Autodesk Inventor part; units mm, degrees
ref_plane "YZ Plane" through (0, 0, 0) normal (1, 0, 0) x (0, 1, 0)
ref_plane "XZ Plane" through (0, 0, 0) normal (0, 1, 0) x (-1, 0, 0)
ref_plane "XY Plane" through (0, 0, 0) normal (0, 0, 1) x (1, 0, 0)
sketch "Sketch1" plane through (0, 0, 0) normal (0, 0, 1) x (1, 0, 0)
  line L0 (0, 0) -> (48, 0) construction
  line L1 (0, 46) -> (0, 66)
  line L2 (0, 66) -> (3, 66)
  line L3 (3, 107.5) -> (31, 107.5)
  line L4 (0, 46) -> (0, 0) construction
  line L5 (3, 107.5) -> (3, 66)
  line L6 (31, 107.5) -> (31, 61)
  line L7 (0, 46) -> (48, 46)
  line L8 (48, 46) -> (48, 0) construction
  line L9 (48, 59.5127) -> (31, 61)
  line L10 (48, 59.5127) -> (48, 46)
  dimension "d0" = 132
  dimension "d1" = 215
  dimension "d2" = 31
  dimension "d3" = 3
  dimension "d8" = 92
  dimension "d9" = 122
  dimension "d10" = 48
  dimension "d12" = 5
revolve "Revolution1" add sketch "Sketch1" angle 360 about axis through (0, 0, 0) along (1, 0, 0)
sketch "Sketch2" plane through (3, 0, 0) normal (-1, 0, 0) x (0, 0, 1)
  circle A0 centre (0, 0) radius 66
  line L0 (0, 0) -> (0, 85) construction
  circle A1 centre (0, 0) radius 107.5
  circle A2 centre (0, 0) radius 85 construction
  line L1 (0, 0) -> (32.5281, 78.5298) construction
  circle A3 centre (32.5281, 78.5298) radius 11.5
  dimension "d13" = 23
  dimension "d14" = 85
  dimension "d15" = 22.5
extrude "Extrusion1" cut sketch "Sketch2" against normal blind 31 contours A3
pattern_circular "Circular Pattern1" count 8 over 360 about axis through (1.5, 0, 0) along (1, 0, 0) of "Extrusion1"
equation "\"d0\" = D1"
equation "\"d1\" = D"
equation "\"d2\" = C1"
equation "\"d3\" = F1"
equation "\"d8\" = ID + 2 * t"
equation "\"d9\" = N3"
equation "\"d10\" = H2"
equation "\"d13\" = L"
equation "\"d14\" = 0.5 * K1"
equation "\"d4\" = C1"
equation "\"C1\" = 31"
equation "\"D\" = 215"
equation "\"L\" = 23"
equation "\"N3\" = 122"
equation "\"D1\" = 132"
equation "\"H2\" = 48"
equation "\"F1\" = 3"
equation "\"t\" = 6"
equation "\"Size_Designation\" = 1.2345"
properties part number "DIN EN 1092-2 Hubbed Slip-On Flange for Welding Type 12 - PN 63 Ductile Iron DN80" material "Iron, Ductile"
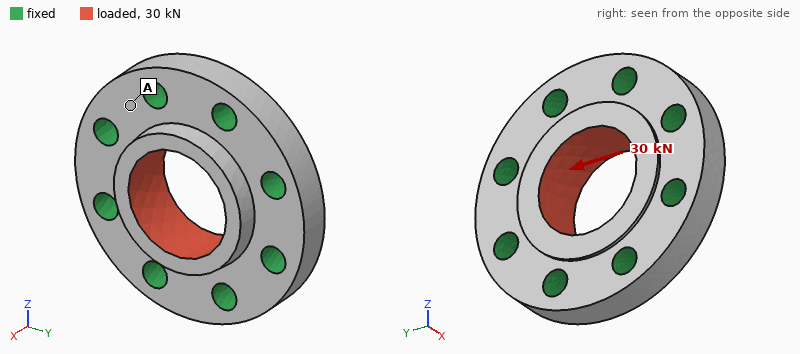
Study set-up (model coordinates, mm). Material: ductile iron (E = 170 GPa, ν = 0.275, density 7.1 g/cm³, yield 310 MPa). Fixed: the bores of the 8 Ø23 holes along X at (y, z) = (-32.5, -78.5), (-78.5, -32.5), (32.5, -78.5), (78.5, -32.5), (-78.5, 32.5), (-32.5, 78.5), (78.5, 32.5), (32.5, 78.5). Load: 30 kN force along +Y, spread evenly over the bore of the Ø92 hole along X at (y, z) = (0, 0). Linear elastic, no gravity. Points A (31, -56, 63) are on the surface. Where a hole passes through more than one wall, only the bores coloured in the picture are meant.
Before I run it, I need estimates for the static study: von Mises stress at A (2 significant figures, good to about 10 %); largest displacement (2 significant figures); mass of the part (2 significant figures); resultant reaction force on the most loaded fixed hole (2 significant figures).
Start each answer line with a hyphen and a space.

- 1.1 MPa
- 2.6 µm
- 6.0 kg
- 5.1 kN
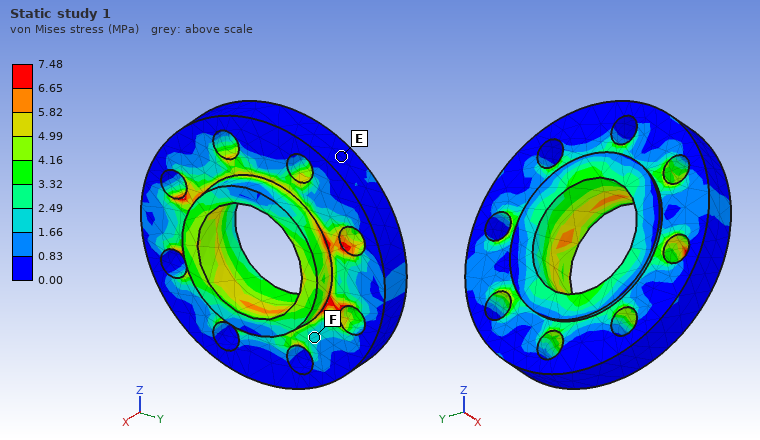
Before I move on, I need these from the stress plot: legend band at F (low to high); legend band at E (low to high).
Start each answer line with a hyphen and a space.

- 1.66 to 2.49 MPa
- 0.00 to 0.83 MPa
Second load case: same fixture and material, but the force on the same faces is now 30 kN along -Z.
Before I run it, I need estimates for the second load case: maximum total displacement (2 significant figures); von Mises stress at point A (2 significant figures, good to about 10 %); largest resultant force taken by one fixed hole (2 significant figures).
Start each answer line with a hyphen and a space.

- 2.5 µm
- 1.2 MPa
- 5.1 kN
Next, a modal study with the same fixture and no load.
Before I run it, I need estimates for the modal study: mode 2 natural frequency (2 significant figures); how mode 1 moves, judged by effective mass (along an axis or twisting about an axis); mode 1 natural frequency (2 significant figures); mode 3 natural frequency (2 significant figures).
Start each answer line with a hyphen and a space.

- 15 kHz
- along X
- 13 kHz
- 15 kHz
